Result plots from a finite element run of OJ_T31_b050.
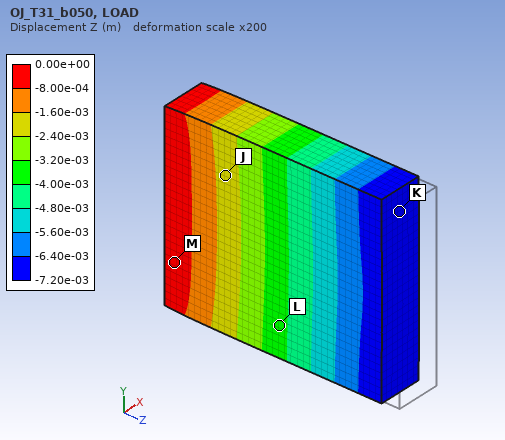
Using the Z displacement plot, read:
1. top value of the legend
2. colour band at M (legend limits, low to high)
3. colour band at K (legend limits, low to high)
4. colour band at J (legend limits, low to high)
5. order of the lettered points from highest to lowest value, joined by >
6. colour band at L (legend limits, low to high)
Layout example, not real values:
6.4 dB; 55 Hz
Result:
0.00e+00 m; -8.00e-04 to 0.00e+00 m; -7.20e-03 to -6.40e-03 m; -2.40e-03 to -1.60e-03 m; M > J > L > K; -4.00e-03 to -3.20e-03 m
